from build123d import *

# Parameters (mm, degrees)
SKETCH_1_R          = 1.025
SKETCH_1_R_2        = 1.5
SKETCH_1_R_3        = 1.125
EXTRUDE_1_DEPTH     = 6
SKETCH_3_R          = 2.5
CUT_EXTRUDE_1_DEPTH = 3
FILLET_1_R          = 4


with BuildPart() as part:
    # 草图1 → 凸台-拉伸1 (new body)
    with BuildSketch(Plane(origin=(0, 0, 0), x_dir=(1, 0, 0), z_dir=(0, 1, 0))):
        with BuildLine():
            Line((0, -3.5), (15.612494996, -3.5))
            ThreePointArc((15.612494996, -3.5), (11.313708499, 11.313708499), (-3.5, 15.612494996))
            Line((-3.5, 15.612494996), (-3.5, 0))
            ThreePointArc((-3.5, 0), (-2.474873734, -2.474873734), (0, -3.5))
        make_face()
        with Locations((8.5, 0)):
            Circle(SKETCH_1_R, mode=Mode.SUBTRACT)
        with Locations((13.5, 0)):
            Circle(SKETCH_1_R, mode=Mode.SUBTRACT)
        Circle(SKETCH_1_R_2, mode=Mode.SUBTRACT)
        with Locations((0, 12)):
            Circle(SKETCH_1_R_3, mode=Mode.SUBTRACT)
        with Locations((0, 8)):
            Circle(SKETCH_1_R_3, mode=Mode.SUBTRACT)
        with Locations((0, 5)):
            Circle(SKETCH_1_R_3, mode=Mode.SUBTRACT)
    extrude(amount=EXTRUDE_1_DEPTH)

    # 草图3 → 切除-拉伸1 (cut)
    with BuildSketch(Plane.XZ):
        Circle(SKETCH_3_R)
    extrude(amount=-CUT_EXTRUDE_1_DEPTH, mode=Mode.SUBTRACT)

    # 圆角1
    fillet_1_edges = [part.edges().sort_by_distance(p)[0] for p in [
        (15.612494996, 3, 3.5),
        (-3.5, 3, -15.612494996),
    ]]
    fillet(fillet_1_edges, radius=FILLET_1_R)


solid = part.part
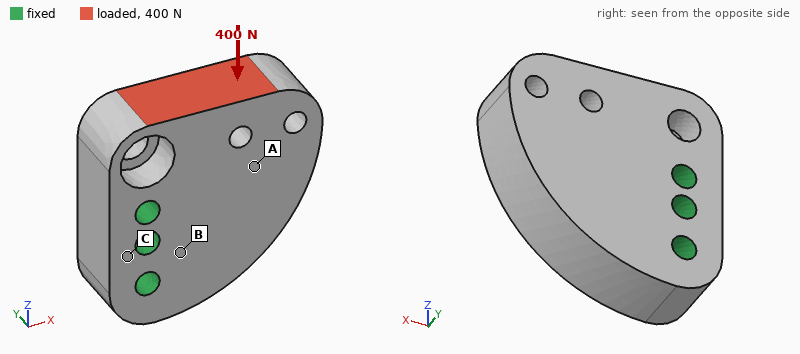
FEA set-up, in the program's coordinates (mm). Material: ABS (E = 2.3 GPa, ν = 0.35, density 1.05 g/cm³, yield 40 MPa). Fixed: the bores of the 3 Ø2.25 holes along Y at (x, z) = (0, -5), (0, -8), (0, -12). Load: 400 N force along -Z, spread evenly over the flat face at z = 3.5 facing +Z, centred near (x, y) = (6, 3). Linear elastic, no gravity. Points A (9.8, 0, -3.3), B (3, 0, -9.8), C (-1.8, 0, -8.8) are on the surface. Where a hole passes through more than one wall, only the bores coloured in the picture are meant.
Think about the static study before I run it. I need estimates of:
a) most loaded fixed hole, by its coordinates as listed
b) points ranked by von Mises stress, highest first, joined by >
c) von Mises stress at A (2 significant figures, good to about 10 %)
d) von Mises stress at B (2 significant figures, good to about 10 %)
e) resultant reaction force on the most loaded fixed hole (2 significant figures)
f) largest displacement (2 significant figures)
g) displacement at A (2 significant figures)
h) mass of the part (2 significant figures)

(0, -5)
B > A > C
5.0 MPa
9.8 MPa
310 N
0.12 mm
0.082 mm
1.8 g
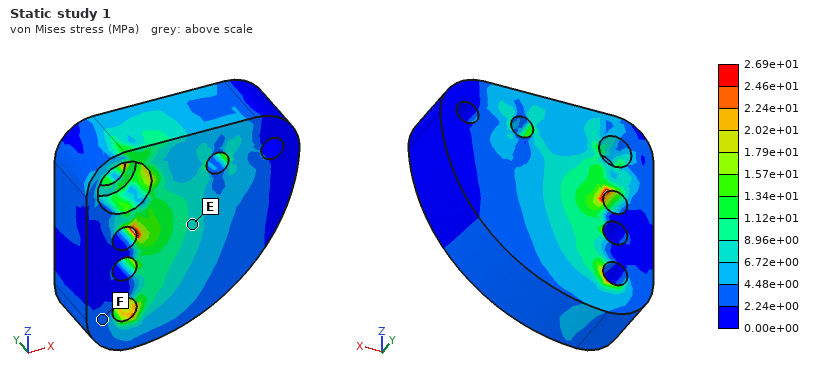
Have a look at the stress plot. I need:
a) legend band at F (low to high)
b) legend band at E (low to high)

2.24e+00 to 4.48e+00 MPa
6.72e+00 to 8.96e+00 MPa
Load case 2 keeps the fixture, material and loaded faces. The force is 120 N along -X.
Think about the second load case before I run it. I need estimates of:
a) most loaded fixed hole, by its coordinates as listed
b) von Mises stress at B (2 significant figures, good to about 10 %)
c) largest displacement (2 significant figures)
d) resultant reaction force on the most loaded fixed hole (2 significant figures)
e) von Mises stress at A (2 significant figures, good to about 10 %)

(0, -5)
2.9 MPa
75 µm
210 N
1.7 MPa
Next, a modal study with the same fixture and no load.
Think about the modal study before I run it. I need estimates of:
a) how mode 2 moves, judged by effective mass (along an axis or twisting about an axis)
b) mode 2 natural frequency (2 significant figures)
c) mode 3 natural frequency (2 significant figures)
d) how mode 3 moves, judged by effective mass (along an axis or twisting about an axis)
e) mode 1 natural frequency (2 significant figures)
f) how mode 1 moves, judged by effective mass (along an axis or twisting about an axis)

along Z
8100 Hz
11 kHz
twisting about X
5600 Hz
along Y
